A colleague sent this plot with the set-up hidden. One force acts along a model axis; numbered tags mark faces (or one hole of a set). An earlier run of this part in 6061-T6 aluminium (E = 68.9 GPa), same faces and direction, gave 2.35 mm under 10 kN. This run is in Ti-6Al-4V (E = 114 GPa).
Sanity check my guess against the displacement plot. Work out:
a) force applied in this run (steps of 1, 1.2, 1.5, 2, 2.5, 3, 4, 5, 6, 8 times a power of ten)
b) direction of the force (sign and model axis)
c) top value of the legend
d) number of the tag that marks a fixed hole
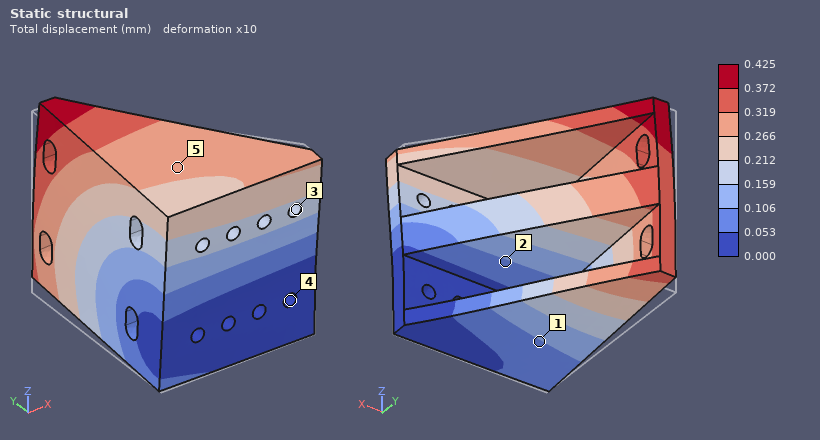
3 kN
-Y
0.425 mm
4
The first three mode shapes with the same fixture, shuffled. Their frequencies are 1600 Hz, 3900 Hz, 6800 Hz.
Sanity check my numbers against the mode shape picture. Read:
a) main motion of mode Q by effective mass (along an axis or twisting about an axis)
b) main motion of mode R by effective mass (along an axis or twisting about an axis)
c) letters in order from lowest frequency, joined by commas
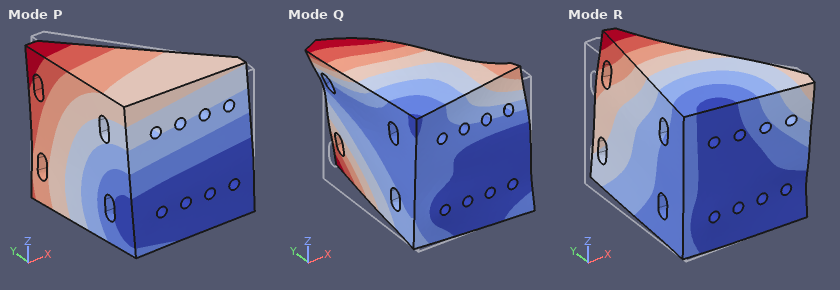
along Y
along X
P, R, Q
